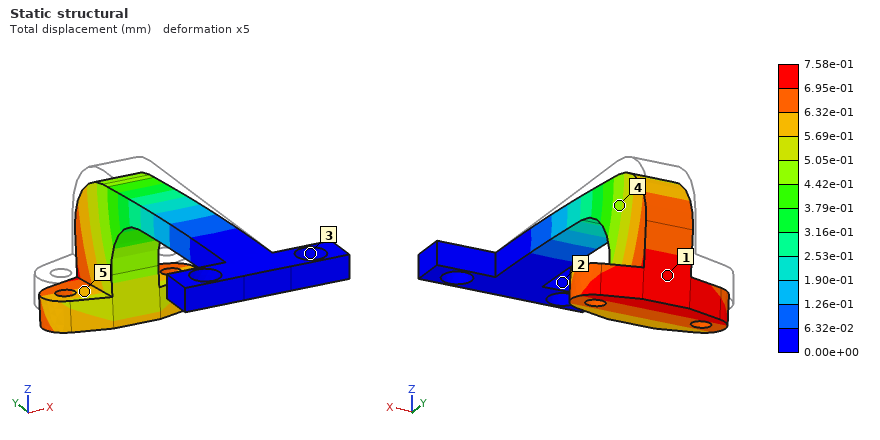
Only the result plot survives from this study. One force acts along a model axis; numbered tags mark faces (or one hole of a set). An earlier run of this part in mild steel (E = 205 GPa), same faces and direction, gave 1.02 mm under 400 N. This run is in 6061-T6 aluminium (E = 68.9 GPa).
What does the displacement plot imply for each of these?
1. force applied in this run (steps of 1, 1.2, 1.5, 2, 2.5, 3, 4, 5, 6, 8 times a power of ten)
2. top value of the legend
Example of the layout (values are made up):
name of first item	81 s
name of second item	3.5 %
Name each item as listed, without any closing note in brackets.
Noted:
force applied in this run	100 N
top value of the legend	7.58e-01 mm
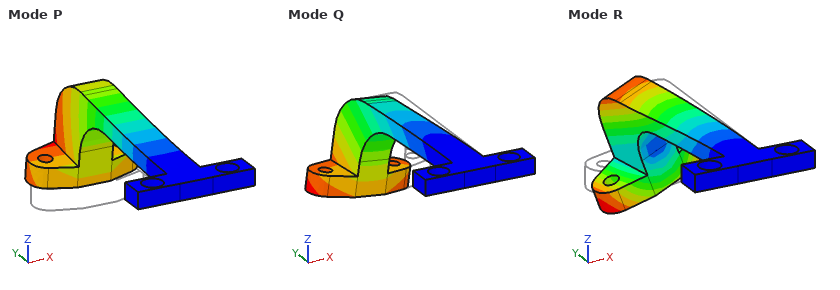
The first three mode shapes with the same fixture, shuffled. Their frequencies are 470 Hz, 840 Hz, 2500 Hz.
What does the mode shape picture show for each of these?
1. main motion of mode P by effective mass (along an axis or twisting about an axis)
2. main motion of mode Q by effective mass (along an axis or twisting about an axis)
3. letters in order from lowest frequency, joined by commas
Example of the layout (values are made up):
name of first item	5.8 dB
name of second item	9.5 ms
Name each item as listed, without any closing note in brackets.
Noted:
main motion of mode P by effective mass	along Z
main motion of mode Q by effective mass	along X
letters in order from lowest frequency, joined by commas	P, Q, R
